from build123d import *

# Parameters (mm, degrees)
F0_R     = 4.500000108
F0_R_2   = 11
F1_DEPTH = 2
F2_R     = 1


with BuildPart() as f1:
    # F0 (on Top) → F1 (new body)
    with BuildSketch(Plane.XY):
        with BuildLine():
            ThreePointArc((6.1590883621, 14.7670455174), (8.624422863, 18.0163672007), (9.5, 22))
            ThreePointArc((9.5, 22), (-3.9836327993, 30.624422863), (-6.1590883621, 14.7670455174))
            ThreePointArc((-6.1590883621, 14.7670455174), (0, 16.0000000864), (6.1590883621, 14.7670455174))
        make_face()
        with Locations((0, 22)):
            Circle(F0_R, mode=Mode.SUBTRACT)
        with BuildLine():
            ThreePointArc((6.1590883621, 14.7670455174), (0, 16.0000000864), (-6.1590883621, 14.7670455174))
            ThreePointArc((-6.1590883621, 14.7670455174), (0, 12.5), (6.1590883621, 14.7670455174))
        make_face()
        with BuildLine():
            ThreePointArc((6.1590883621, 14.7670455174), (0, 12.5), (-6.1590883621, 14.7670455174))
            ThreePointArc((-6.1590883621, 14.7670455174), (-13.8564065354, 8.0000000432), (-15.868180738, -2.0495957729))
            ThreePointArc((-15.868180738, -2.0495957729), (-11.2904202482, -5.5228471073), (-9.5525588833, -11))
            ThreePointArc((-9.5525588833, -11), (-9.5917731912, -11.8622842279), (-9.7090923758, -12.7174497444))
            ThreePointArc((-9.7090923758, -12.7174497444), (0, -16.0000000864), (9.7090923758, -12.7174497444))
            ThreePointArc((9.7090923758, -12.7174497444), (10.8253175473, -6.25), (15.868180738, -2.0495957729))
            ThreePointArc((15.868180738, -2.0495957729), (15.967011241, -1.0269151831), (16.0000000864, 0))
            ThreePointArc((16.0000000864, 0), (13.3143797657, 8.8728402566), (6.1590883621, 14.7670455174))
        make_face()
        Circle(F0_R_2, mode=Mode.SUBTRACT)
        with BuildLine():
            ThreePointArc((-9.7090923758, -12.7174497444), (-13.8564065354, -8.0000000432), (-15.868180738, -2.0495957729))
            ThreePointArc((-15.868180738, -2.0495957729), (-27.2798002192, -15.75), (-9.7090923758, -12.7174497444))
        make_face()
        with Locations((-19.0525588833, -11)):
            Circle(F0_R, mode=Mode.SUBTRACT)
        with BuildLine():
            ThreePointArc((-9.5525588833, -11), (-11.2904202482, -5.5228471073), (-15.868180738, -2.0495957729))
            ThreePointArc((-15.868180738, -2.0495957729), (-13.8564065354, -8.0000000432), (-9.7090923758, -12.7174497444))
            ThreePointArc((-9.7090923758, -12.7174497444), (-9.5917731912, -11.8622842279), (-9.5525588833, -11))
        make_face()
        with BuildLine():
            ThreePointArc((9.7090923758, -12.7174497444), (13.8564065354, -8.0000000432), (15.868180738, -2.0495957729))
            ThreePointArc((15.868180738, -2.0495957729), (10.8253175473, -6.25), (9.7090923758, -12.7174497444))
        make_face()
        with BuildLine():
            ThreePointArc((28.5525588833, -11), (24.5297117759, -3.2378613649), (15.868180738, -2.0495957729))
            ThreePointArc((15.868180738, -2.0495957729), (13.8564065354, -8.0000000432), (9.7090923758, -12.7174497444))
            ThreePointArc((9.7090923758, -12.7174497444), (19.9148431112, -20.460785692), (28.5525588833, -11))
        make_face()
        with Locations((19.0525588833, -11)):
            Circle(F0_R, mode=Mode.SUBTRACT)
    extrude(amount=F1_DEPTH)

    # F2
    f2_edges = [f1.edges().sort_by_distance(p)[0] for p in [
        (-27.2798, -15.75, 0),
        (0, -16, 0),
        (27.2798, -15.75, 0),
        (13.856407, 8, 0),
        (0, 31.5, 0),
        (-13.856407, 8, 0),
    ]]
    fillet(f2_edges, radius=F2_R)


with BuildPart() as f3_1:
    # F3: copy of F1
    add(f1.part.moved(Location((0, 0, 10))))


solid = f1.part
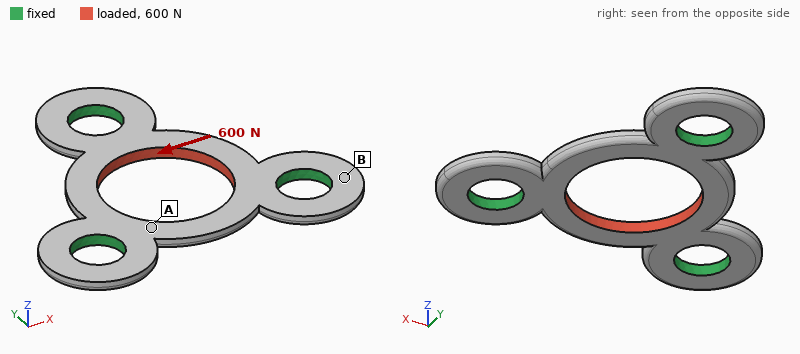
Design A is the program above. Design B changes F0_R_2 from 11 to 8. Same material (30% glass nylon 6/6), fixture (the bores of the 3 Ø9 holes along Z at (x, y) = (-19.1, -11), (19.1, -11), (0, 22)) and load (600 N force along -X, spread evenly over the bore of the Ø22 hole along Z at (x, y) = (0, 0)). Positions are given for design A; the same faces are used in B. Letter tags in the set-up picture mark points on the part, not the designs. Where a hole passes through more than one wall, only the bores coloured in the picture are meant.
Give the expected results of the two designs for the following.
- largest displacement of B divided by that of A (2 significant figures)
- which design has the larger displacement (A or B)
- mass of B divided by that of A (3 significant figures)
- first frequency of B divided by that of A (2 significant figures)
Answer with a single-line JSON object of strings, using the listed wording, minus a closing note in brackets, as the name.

{"largest displacement of B divided by that of A": "0.81", "which design has the larger displacement": "A", "mass of B divided by that of A": "1.18", "first frequency of B divided by that of A": "0.91"}
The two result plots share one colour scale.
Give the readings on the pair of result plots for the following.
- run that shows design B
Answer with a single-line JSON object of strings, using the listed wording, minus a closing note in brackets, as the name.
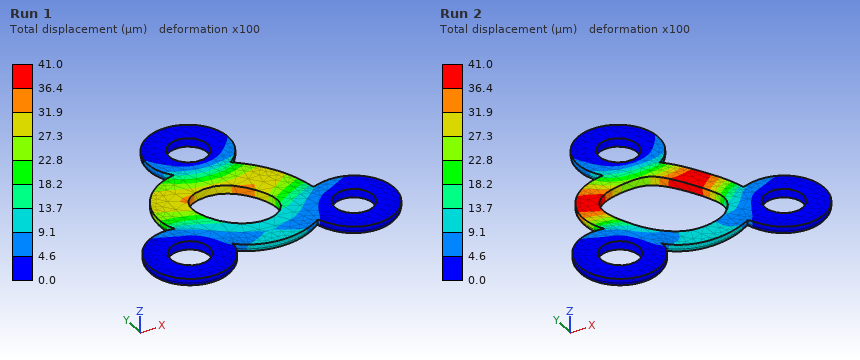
{"run that shows design B": "Run 1"}
